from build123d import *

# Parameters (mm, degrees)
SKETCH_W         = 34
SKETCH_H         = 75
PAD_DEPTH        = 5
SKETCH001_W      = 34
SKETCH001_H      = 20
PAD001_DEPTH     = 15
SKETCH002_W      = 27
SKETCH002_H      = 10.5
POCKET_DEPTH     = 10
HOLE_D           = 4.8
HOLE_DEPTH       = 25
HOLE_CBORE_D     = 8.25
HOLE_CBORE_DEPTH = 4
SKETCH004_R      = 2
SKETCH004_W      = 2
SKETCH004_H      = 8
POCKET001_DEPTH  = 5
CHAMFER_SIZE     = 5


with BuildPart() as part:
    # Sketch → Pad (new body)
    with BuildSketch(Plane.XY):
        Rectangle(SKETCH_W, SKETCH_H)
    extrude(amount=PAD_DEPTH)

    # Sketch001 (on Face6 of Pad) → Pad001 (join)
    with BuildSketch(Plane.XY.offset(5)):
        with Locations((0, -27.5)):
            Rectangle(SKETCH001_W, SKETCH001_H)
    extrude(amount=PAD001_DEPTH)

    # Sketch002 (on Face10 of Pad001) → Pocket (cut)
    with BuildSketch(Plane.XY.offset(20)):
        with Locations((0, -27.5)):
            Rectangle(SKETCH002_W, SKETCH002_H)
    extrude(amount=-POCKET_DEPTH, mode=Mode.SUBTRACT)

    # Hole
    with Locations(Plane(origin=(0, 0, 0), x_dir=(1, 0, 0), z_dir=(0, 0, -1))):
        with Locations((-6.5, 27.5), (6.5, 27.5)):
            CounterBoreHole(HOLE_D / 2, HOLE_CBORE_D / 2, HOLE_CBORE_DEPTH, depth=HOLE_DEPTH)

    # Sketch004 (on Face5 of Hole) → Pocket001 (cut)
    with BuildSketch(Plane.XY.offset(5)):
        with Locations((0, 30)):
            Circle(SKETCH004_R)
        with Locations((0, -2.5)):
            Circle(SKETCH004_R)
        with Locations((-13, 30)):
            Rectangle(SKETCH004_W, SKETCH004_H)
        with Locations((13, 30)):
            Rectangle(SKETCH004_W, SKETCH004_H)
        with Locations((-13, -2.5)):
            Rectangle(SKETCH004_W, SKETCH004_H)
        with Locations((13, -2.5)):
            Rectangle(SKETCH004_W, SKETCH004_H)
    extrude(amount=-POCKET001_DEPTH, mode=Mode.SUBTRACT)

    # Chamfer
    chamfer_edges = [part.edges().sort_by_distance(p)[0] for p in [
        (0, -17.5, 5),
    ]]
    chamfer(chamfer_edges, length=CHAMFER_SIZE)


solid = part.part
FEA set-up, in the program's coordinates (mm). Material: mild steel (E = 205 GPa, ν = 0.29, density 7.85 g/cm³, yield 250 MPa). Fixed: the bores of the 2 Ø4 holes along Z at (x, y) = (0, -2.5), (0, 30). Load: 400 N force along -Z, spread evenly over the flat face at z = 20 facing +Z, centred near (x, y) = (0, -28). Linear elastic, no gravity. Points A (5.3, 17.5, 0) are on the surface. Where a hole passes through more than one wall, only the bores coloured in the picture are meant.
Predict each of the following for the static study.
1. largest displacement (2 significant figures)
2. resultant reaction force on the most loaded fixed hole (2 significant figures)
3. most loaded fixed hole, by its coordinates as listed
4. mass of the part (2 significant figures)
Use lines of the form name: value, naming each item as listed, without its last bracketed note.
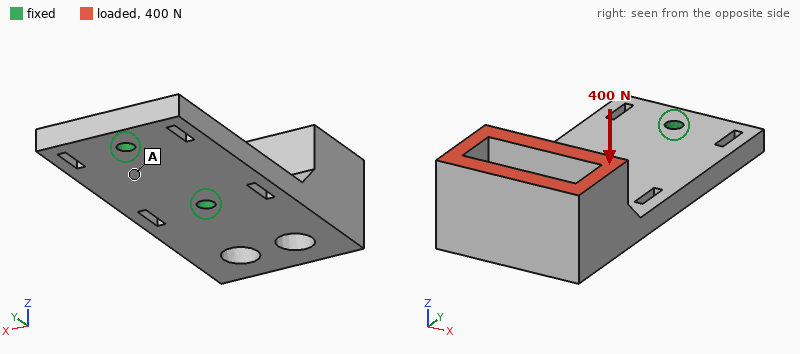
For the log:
largest displacement: 57 µm
resultant reaction force on the most loaded fixed hole: 500 N
most loaded fixed hole, by its coordinates as listed: (0, -2.5)
mass of the part: 150 g
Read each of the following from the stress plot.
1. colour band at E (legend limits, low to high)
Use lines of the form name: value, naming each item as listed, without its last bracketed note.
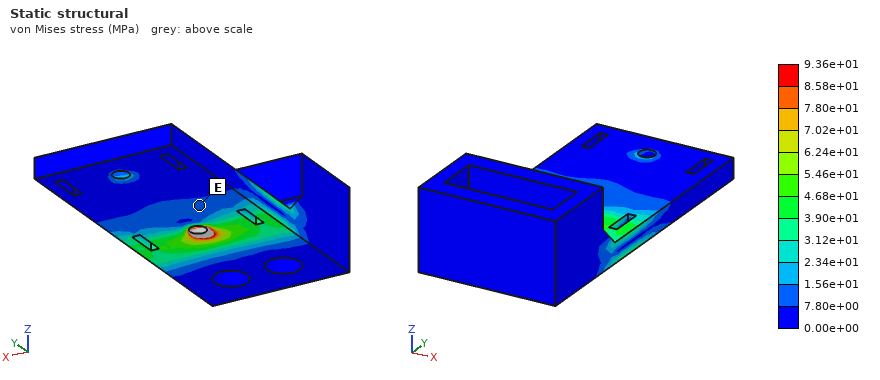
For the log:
colour band at E: 7.80e+00 to 1.56e+01 MPa
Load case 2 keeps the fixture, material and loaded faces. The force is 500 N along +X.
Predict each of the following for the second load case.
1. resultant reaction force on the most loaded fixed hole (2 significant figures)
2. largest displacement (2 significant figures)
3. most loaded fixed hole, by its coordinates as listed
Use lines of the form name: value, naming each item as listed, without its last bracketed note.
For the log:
resultant reaction force on the most loaded fixed hole: 830 N
largest displacement: 31 µm
most loaded fixed hole, by its coordinates as listed: (0, -2.5)
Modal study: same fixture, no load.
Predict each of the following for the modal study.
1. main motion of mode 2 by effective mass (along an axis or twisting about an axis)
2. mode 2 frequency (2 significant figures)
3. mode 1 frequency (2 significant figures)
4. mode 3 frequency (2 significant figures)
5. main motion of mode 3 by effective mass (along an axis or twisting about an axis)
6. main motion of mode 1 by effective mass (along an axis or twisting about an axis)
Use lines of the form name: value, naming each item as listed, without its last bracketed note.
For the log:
main motion of mode 2 by effective mass: along X
mode 2 frequency: 3400 Hz
mode 1 frequency: 1700 Hz
mode 3 frequency: 6300 Hz
main motion of mode 3 by effective mass: along X
main motion of mode 1 by effective mass: along Z
